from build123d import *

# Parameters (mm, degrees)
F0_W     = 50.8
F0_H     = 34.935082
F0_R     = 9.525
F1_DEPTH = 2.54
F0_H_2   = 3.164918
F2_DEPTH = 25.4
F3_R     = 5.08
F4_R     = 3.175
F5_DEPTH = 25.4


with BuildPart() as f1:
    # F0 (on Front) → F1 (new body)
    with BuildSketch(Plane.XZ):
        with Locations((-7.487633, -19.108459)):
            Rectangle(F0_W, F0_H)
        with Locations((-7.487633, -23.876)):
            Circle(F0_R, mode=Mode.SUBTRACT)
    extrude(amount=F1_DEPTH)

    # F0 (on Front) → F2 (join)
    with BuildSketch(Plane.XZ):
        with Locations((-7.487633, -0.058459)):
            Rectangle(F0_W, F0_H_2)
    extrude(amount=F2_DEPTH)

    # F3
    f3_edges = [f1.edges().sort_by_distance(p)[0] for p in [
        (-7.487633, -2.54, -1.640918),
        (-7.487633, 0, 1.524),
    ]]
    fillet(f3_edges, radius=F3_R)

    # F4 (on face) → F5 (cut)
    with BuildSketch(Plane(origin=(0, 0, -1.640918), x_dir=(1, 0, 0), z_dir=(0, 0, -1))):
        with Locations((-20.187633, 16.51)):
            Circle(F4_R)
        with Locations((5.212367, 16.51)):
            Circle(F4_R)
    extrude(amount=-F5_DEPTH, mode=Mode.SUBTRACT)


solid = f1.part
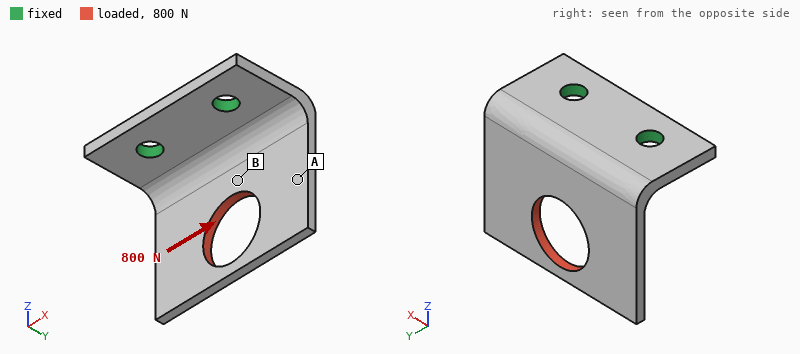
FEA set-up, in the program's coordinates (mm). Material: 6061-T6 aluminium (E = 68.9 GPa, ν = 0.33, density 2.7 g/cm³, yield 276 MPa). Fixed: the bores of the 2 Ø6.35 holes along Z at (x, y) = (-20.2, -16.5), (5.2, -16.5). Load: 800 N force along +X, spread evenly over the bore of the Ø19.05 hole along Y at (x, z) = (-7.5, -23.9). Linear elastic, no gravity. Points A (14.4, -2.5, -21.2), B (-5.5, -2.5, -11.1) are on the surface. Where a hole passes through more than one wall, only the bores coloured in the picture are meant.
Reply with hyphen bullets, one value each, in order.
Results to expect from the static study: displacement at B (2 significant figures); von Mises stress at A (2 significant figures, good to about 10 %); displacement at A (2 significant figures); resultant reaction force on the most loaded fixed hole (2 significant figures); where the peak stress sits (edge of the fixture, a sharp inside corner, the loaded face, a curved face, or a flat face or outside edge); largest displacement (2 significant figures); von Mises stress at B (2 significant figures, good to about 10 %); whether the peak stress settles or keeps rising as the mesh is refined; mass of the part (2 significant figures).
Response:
- 0.058 mm
- 25 MPa
- 0.18 mm
- 830 N
- edge of the fixture
- 0.28 mm
- 58 MPa
- keeps rising
- 21 g
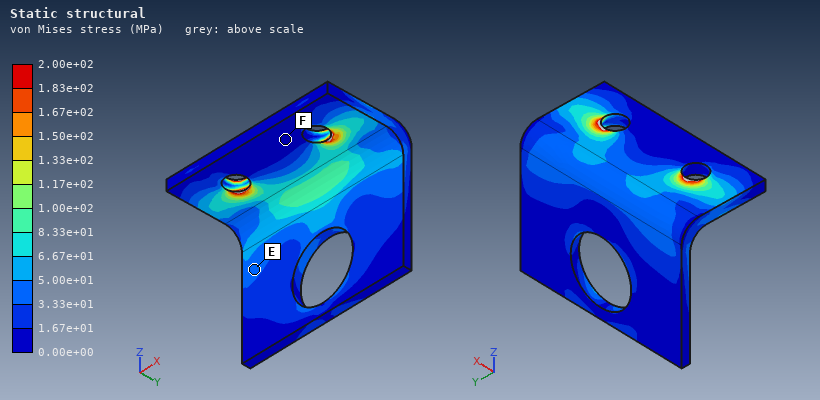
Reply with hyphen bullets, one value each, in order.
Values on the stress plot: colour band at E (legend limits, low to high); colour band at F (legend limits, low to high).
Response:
- 3.33e+01 to 5.00e+01 MPa
- 0.00e+00 to 1.67e+01 MPa
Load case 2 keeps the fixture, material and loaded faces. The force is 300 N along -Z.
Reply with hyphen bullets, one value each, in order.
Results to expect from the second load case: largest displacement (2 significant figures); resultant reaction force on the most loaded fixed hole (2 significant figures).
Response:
- 0.11 mm
- 150 N
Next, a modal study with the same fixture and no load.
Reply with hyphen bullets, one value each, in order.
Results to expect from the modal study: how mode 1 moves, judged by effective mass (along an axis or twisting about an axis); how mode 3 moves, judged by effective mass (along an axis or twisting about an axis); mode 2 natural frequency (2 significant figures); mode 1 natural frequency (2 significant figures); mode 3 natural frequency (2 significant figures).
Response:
- along Y
- along X
- 2500 Hz
- 1500 Hz
- 4100 Hz
